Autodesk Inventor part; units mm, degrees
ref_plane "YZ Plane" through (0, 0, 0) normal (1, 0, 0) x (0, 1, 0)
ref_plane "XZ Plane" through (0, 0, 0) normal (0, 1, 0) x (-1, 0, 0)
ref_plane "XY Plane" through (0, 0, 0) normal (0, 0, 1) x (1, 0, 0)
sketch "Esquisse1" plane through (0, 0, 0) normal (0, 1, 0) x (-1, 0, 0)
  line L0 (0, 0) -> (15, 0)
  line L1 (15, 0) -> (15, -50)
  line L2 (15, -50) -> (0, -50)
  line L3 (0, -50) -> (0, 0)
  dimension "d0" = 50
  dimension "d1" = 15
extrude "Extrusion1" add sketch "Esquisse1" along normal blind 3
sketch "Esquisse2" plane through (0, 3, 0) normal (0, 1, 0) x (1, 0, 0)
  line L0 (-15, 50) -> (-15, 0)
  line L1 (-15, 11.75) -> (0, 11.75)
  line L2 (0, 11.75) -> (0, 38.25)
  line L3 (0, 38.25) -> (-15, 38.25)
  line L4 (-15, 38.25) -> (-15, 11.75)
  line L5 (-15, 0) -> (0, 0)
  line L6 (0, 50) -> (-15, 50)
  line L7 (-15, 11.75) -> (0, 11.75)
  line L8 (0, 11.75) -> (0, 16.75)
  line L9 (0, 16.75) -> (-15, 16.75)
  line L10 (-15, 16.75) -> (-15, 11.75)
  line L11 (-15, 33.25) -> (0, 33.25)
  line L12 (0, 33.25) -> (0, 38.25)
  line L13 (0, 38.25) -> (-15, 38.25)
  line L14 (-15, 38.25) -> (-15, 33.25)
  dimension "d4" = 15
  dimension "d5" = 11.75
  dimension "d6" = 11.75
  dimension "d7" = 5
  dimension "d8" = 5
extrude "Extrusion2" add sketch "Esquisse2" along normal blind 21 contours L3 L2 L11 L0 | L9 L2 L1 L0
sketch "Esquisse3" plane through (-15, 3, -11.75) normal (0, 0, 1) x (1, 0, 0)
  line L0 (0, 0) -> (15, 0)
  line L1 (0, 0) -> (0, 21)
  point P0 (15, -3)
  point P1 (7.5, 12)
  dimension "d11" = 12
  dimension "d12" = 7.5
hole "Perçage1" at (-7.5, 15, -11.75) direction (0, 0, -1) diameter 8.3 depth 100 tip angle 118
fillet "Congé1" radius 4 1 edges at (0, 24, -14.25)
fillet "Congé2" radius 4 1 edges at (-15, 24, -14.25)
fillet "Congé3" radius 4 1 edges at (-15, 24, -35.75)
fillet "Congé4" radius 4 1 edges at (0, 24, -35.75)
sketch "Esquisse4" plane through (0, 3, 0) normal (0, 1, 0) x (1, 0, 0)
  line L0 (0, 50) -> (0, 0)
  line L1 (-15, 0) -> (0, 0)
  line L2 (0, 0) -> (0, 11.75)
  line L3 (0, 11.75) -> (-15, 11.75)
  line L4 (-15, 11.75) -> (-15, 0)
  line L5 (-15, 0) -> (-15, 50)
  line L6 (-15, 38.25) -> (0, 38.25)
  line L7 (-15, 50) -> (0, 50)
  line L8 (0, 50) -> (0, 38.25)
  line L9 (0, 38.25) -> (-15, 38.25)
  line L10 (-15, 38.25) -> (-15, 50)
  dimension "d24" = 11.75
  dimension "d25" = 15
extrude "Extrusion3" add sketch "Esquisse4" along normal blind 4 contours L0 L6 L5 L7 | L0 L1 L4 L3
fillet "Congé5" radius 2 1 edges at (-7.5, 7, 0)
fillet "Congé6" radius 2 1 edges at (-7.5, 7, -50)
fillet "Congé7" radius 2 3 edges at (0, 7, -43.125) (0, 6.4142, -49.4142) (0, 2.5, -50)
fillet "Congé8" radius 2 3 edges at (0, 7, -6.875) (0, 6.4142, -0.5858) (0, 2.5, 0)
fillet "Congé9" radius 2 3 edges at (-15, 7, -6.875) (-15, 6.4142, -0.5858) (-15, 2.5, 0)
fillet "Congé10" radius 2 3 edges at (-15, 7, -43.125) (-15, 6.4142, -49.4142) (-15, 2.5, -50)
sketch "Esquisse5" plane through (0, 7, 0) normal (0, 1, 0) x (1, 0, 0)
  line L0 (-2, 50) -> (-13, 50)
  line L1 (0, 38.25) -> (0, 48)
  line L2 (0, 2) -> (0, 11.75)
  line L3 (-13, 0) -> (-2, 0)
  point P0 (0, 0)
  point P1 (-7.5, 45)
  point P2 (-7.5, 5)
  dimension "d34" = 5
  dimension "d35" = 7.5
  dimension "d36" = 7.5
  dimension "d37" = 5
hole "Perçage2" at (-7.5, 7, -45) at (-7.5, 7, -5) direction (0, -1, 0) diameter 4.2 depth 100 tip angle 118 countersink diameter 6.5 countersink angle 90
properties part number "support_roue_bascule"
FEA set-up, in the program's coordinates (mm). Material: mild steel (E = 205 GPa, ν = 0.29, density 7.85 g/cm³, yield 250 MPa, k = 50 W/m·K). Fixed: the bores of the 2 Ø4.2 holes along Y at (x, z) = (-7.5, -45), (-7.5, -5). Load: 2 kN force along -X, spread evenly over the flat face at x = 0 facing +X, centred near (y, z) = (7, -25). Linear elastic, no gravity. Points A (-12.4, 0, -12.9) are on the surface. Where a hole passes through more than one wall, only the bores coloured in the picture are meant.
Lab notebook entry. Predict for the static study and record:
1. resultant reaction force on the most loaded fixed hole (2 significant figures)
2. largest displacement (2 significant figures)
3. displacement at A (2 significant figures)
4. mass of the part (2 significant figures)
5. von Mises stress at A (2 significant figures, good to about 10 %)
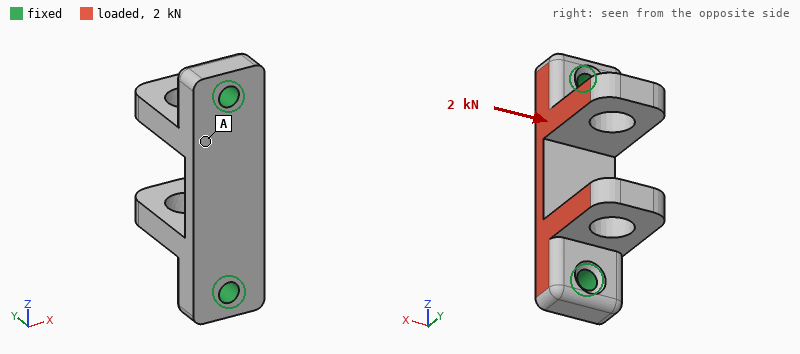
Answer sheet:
1.0 kN
11 µm
1.9 µm
46 g
12 MPa
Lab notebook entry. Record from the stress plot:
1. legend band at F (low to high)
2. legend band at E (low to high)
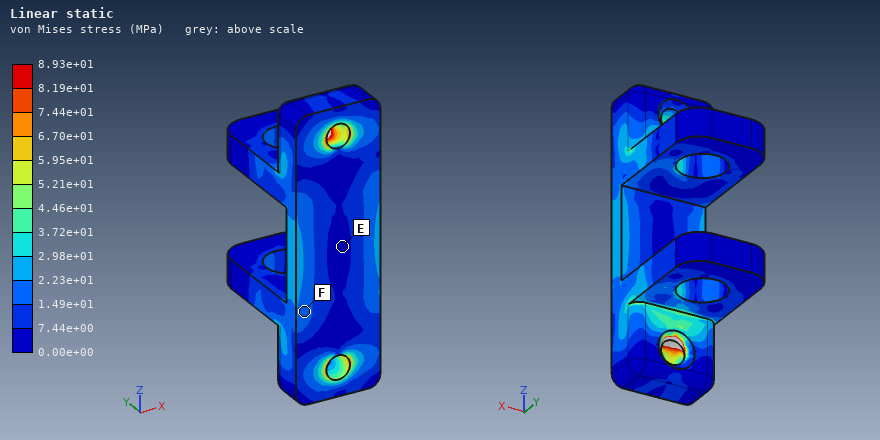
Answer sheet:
1.49e+01 to 2.23e+01 MPa
0.00e+00 to 7.44e+00 MPa
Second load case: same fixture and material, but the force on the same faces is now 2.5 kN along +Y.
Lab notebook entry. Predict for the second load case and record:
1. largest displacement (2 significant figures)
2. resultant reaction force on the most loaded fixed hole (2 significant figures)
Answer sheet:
23 µm
1.3 kN
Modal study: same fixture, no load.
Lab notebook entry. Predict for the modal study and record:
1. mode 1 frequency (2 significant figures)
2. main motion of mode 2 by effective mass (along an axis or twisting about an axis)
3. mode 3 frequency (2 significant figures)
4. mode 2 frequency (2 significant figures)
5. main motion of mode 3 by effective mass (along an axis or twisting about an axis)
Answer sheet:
8300 Hz
along Z
11 kHz
8900 Hz
along X
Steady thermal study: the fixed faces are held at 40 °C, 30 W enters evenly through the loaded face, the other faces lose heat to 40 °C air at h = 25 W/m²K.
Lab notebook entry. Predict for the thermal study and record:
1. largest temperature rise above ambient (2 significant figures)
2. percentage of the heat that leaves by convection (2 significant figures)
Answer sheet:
44 K
5.6 %
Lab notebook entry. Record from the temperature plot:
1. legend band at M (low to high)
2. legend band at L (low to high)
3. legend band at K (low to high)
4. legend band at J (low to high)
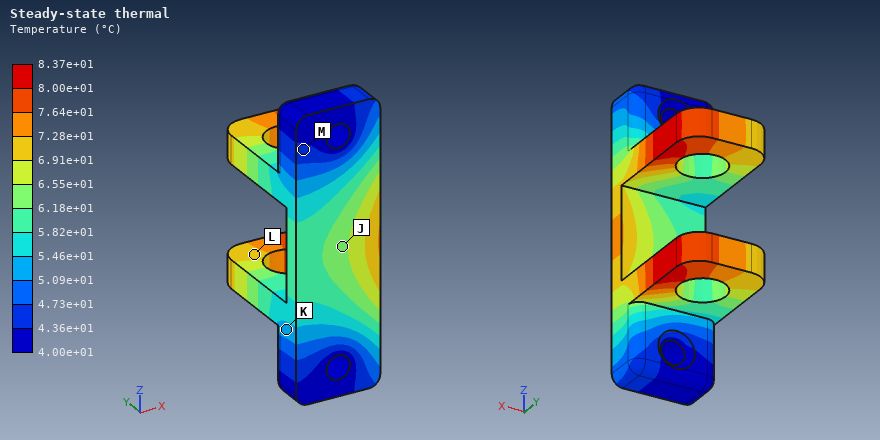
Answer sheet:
4.36e+01 to 4.73e+01 °C
6.91e+01 to 7.28e+01 °C
5.09e+01 to 5.46e+01 °C
6.18e+01 to 6.55e+01 °C
